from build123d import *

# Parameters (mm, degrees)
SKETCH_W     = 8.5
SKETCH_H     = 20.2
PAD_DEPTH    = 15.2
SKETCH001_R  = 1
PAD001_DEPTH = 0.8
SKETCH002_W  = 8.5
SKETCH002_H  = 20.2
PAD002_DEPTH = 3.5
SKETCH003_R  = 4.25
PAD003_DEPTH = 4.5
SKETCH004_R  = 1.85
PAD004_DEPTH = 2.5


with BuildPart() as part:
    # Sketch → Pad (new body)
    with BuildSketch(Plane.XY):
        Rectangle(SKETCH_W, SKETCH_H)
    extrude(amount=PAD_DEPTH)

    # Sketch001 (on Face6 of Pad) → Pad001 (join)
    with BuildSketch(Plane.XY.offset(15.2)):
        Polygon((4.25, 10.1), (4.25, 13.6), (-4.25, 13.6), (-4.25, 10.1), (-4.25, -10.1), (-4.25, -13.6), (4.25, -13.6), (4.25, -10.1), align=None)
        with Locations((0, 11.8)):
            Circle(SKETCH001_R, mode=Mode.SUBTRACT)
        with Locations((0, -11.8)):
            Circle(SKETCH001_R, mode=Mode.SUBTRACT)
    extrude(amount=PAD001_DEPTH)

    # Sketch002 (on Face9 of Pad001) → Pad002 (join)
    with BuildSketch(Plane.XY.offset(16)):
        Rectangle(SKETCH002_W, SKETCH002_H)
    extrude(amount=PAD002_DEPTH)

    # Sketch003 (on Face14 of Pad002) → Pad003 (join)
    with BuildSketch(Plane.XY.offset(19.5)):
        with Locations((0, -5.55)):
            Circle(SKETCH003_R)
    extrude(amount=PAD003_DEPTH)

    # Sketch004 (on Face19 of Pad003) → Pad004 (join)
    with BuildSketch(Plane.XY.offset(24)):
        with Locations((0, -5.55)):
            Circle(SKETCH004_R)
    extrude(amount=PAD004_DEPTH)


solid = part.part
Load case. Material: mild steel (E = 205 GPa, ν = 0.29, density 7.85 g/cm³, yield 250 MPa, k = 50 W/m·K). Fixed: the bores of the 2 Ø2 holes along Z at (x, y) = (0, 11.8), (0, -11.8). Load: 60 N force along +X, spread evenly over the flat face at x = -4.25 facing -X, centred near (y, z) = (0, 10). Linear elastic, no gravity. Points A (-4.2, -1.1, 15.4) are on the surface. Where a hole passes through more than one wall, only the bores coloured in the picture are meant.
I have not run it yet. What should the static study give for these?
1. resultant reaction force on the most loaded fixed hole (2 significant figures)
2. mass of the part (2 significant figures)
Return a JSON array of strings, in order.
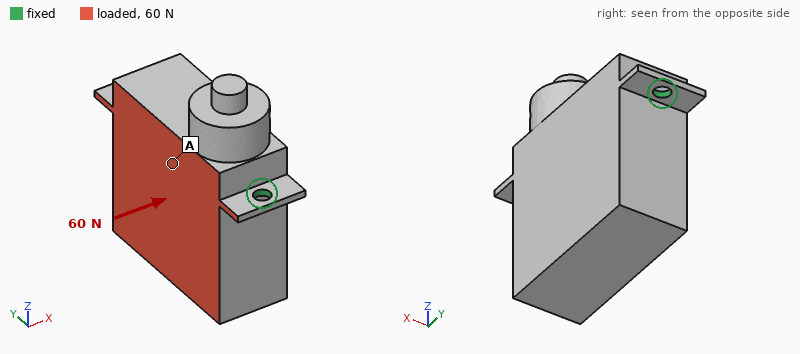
["30 N", "29 g"]
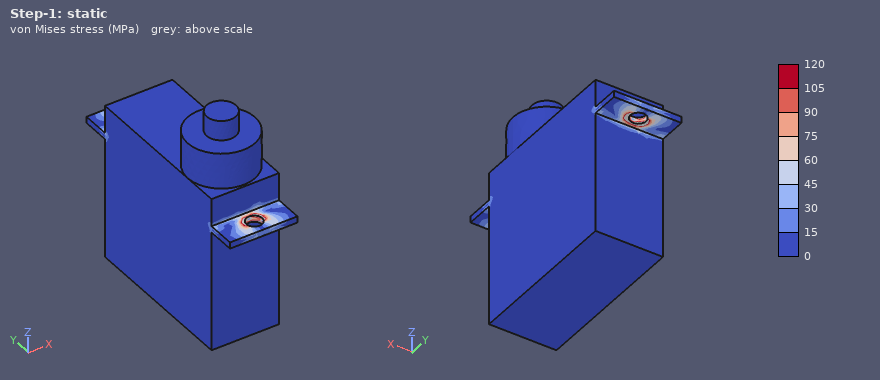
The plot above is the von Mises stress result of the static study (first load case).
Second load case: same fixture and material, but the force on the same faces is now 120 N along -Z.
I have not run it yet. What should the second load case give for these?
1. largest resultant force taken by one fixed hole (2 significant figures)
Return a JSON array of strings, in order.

["60 N"]
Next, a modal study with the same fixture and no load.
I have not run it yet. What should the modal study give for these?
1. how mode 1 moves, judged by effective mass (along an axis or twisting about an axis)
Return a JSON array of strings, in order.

["along X"]
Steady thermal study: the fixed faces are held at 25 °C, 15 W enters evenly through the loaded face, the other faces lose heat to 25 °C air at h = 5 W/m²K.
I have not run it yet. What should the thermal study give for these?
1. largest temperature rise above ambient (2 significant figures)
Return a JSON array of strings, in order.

["69 K"]
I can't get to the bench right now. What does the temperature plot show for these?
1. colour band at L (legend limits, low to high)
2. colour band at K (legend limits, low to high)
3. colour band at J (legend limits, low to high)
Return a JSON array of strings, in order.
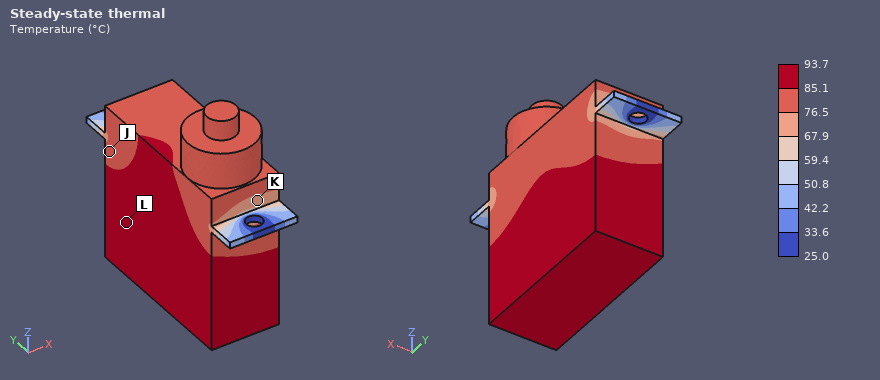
["85.1 to 93.7 °C", "67.9 to 76.5 °C", "76.5 to 85.1 °C"]
